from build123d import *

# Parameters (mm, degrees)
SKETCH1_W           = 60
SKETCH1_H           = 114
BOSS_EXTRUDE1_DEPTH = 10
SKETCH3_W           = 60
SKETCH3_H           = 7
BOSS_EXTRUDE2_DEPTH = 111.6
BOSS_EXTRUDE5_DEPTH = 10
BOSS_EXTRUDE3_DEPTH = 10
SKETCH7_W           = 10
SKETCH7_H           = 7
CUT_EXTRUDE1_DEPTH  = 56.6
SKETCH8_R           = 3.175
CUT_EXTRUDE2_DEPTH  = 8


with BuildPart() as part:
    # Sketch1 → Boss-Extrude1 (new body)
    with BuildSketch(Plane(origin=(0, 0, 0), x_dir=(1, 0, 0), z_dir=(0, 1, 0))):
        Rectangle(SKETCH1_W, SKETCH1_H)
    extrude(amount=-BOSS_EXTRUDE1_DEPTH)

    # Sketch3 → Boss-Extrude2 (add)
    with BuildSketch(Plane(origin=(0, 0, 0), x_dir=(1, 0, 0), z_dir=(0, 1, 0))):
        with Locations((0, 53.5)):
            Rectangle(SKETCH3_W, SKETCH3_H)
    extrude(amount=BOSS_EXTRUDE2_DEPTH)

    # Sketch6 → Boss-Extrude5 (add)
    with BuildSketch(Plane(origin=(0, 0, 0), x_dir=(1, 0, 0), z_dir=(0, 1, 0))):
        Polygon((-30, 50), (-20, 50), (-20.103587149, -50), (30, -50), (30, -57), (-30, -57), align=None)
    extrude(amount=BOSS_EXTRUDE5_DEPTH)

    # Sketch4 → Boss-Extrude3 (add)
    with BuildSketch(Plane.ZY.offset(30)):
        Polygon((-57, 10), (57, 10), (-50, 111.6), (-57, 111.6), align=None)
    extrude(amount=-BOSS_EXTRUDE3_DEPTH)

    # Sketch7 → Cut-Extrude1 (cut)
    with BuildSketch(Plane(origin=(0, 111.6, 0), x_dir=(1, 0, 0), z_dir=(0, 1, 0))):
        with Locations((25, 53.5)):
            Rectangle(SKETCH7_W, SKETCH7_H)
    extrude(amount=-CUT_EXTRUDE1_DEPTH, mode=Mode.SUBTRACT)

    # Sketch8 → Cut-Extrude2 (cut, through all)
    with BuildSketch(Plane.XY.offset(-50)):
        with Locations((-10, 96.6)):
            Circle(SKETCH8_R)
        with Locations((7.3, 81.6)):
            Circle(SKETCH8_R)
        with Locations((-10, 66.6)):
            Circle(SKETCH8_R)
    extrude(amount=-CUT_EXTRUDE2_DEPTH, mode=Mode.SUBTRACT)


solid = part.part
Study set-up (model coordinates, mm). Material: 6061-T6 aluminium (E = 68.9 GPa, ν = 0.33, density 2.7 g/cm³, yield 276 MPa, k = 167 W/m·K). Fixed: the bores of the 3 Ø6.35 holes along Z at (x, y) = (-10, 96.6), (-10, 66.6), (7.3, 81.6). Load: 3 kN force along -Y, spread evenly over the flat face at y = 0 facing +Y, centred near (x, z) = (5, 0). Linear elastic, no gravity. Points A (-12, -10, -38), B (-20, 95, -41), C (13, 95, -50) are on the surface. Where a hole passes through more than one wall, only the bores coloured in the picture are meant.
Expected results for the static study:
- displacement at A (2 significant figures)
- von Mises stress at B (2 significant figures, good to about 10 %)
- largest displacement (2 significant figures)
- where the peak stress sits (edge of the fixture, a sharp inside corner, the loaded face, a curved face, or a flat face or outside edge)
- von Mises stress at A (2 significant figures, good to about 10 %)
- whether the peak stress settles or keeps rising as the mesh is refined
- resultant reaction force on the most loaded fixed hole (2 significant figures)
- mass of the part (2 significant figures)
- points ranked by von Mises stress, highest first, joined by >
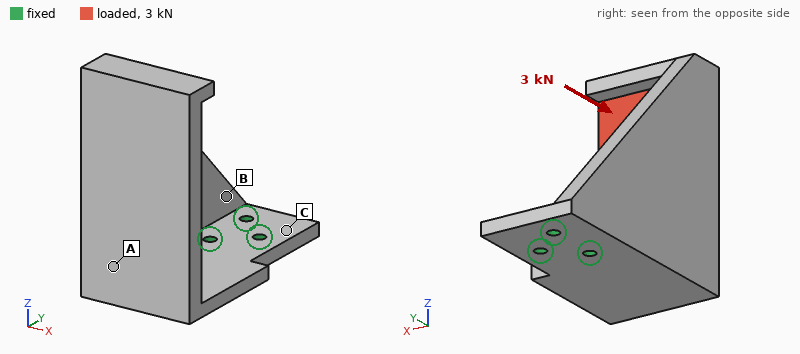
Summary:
0.30 mm
70 MPa
0.81 mm
edge of the fixture
28 MPa
keeps rising
4.6 kN
480 g
B > A > C
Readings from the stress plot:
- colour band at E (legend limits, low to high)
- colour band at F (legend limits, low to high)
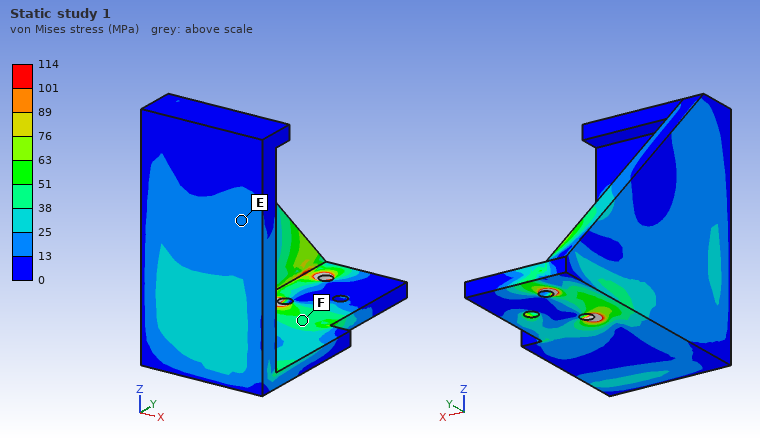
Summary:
13 to 25 MPa
38 to 51 MPa
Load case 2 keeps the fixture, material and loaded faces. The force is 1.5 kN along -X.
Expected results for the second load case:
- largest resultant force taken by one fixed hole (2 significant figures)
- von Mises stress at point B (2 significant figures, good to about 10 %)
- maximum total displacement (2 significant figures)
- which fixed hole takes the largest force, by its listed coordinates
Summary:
3.5 kN
50 MPa
1.4 mm
(-10, 66.6)
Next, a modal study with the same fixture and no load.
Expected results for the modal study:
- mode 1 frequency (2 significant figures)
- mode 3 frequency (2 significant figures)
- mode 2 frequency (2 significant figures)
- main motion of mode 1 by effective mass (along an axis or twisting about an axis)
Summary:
360 Hz
1600 Hz
650 Hz
along X
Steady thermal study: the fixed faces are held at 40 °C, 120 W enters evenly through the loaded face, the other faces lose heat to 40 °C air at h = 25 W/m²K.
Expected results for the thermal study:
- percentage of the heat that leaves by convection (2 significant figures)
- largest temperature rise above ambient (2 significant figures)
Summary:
32 %
71 K
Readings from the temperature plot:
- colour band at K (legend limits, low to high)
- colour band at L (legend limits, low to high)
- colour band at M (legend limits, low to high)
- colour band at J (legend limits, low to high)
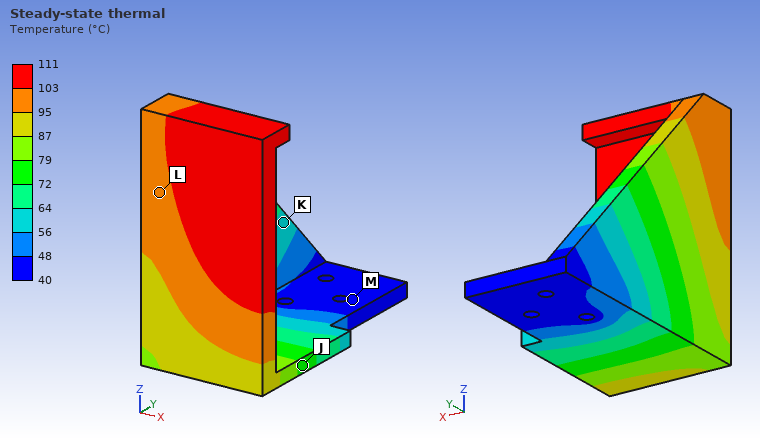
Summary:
56 to 64 °C
95 to 103 °C
40 to 48 °C
72 to 79 °C
